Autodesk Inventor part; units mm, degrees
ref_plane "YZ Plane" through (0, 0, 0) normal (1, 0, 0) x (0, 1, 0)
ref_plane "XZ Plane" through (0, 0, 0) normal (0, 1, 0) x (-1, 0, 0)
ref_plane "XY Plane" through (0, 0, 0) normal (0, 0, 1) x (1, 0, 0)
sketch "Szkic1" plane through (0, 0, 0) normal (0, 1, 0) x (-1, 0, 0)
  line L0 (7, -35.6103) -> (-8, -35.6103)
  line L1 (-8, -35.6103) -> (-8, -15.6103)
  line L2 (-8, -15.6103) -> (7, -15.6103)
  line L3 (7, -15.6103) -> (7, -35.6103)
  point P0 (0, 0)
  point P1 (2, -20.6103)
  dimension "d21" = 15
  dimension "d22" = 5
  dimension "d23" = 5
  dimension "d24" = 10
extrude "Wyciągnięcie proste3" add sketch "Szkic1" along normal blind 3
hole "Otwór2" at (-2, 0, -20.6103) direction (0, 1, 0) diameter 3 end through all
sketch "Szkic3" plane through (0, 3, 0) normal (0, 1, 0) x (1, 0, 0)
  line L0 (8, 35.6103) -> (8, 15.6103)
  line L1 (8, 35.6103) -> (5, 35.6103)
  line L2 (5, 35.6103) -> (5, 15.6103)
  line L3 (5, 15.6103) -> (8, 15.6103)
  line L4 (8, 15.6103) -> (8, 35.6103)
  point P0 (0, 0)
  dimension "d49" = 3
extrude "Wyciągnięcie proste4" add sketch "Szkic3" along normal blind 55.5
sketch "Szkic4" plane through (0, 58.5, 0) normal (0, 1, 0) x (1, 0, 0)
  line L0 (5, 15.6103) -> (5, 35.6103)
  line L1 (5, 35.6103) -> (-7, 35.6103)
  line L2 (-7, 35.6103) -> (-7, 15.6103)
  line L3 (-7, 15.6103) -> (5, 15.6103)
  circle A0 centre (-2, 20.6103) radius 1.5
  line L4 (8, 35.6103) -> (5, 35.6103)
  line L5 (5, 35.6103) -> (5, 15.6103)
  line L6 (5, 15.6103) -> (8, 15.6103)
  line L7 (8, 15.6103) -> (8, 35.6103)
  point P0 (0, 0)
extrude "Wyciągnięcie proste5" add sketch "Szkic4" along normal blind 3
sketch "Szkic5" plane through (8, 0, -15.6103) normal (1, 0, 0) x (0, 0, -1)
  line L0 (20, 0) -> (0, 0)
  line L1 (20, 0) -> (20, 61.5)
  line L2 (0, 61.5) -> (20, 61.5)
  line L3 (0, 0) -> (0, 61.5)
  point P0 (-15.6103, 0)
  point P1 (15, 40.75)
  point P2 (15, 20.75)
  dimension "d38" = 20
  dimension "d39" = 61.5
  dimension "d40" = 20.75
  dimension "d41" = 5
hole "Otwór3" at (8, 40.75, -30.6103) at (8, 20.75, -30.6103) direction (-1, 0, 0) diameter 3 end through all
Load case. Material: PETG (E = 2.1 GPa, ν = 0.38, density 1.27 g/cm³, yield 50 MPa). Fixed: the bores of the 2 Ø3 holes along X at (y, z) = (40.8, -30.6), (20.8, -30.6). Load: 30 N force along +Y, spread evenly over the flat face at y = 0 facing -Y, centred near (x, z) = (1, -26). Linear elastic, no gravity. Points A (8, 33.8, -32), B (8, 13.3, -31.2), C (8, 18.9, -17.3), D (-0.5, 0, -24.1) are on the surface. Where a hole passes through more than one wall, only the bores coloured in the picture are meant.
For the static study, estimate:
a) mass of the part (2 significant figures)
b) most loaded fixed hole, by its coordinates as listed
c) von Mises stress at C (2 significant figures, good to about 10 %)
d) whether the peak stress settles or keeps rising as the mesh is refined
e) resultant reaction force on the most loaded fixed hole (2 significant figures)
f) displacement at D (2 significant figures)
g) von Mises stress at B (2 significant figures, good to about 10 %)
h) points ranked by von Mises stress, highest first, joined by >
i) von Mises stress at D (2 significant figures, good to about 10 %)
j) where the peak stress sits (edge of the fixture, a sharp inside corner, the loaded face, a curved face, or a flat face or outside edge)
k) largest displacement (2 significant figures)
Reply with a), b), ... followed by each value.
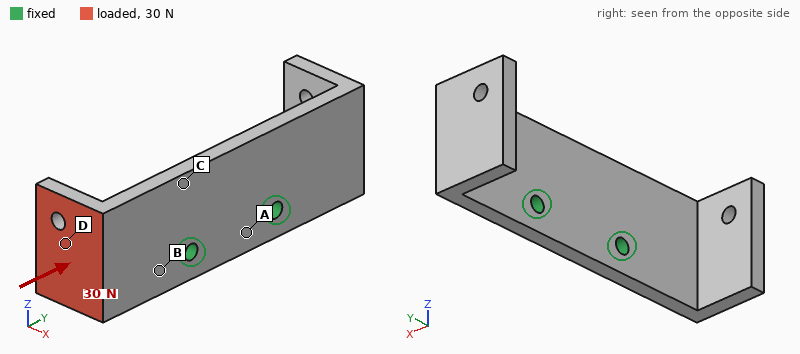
a) 6.4 g
b) (20.8, -30.6)
c) 3.6 MPa
d) keeps rising
e) 23 N
f) 0.51 mm
g) 5.5 MPa
h) B > C > D > A
i) 1.5 MPa
j) edge of the fixture
k) 0.71 mm
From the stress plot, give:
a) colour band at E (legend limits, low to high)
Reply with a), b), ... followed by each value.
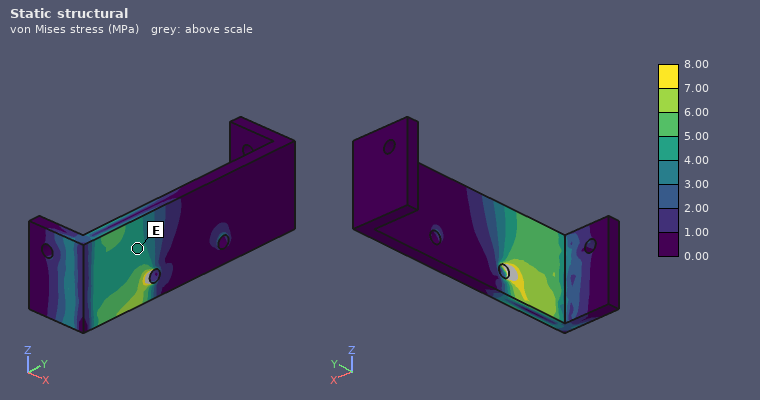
a) 4.00 to 5.00 MPa
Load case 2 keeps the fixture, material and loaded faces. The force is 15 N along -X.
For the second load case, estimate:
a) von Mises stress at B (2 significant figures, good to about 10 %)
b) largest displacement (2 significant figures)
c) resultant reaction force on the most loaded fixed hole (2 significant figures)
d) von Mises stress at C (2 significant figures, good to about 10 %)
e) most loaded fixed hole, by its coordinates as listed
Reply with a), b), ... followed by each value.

a) 7.1 MPa
b) 0.78 mm
c) 20 N
d) 5.5 MPa
e) (20.8, -30.6)
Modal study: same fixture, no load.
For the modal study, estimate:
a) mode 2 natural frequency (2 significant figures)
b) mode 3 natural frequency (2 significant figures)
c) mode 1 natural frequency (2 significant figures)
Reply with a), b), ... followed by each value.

a) 710 Hz
b) 1200 Hz
c) 700 Hz
